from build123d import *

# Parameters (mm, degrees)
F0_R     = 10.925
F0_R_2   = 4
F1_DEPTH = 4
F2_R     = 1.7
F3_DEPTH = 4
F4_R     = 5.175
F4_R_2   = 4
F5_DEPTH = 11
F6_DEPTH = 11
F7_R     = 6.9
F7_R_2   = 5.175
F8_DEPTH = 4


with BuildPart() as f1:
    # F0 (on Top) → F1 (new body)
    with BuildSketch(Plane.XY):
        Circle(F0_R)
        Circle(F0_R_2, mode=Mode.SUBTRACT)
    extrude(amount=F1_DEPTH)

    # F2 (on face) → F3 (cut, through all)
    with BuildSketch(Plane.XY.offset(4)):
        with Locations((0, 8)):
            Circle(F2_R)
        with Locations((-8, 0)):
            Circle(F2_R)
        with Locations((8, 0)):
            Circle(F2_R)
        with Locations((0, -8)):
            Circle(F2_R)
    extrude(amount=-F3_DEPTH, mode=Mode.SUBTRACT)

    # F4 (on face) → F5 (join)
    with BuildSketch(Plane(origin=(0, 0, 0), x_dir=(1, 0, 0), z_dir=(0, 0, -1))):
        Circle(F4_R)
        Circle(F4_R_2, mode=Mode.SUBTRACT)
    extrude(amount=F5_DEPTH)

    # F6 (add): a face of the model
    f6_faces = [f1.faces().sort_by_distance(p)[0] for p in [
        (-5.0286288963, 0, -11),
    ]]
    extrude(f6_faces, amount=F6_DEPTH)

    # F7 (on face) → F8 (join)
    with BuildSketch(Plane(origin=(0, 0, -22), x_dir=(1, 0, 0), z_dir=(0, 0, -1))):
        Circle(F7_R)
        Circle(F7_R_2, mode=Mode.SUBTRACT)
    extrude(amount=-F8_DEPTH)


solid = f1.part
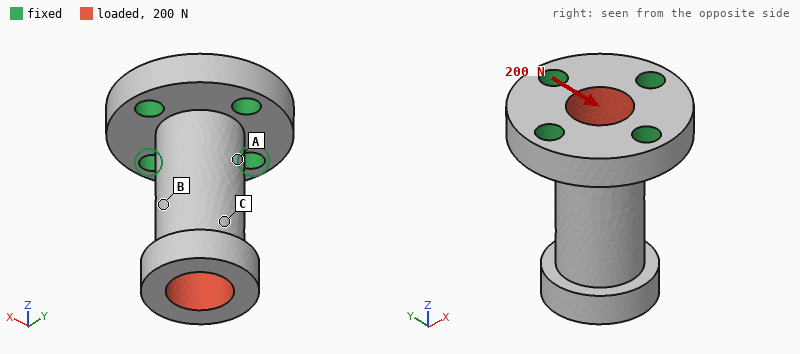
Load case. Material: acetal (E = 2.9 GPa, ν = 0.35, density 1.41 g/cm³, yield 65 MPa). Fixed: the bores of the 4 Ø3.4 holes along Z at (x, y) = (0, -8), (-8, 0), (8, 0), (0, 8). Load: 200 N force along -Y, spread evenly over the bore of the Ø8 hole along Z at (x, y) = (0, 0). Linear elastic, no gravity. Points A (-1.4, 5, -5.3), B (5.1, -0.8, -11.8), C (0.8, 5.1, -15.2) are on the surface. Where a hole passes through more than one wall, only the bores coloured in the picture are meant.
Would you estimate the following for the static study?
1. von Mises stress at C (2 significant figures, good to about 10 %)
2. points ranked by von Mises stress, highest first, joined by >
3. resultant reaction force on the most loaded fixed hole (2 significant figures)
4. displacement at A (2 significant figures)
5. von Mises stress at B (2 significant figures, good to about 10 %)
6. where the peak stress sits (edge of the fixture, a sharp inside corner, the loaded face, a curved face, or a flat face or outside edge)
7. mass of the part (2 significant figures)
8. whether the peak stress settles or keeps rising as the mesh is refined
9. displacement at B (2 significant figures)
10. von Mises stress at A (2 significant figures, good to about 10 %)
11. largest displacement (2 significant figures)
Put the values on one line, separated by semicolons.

2.8 MPa; A > B > C; 170 N; 0.11 mm; 7.3 MPa; a sharp inside corner; 3.0 g; keeps rising; 0.21 mm; 14 MPa; 0.43 mm
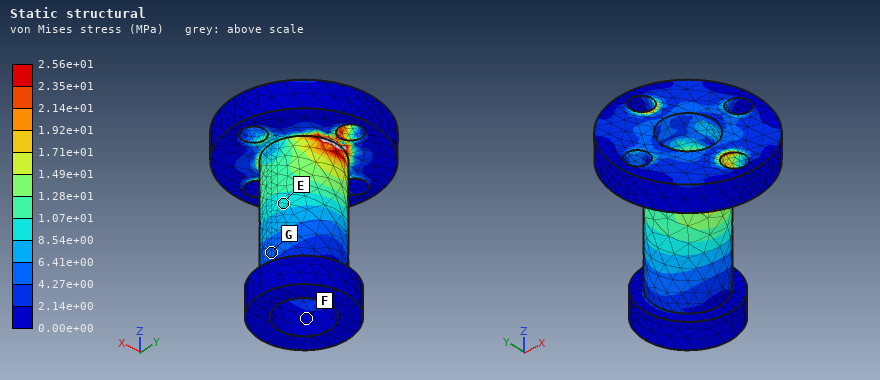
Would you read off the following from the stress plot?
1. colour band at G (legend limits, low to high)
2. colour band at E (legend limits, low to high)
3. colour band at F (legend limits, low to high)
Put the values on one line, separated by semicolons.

4.27e+00 to 6.41e+00 MPa; 8.54e+00 to 1.07e+01 MPa; 0.00e+00 to 2.14e+00 MPa
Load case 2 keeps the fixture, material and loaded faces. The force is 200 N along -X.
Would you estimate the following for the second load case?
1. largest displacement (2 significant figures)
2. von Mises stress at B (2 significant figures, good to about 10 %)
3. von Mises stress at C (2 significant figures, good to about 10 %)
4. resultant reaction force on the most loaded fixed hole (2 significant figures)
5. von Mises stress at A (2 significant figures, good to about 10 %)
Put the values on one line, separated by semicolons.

0.43 mm; 6.0 MPa; 4.9 MPa; 170 N; 12 MPa
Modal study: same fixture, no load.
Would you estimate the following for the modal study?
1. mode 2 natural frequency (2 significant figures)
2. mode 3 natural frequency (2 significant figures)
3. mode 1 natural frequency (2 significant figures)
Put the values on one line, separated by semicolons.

2700 Hz; 6400 Hz; 2700 Hz
